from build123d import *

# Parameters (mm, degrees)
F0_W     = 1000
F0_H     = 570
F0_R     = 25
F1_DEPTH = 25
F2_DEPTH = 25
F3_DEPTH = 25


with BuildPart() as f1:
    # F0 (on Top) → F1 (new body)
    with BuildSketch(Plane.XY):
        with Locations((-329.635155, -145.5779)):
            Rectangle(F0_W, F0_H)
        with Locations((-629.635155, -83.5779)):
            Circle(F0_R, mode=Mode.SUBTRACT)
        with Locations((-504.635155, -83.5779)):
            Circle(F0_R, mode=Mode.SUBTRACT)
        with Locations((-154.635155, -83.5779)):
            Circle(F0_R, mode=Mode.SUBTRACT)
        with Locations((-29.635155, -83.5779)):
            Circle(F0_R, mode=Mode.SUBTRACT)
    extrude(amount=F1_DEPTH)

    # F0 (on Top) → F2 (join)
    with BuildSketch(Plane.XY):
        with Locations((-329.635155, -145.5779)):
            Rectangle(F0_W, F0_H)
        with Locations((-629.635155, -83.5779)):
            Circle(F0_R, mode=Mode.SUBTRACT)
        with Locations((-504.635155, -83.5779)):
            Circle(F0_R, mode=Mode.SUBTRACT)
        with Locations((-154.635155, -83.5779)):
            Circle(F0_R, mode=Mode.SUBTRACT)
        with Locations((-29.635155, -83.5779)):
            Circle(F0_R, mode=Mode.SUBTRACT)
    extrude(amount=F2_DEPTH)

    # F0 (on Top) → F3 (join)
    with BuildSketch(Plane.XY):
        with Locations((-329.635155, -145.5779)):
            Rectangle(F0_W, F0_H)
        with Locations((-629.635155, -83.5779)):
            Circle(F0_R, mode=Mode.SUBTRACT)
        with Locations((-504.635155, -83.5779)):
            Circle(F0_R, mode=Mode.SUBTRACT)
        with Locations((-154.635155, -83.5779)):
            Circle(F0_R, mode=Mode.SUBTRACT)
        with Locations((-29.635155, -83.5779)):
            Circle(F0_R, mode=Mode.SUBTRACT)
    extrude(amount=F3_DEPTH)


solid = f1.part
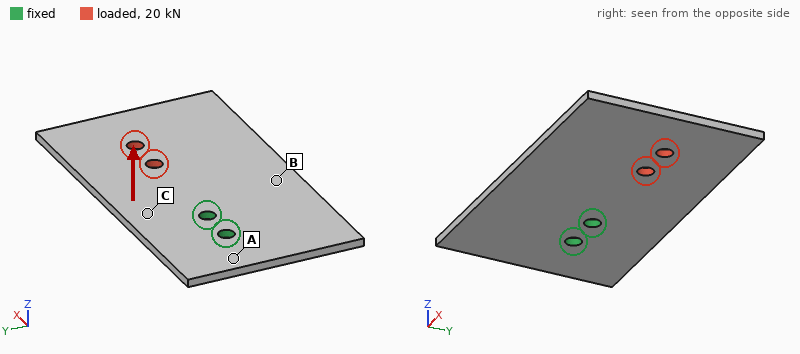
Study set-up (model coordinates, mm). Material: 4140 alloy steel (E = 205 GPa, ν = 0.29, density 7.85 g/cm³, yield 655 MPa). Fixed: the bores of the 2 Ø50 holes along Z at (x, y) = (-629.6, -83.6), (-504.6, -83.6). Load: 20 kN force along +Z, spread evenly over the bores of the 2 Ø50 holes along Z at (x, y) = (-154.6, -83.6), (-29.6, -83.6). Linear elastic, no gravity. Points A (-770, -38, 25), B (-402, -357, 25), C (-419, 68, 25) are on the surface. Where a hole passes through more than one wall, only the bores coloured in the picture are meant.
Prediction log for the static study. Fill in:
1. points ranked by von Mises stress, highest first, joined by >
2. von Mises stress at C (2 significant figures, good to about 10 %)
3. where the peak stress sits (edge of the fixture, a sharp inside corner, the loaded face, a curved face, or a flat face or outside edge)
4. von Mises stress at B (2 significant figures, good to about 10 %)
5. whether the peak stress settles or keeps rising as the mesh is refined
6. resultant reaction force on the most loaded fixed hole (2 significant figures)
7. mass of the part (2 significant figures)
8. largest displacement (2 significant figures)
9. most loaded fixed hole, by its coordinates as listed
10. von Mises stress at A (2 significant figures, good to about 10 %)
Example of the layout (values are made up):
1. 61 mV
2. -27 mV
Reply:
1. C > B > A
2. 110 MPa
3. edge of the fixture
4. 72 MPa
5. keeps rising
6. 45 kN
7. 110 kg
8. 6.9 mm
9. (-504.6, -83.6)
10. 21 MPa
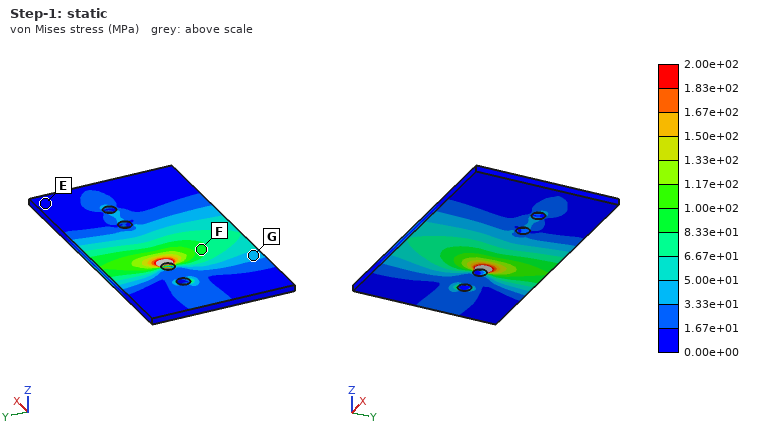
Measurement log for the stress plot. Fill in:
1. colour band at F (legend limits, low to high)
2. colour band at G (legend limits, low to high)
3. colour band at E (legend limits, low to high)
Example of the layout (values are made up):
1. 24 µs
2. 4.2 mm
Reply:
1. 8.33e+01 to 1.00e+02 MPa
2. 3.33e+01 to 5.00e+01 MPa
3. 0.00e+00 to 1.67e+01 MPa
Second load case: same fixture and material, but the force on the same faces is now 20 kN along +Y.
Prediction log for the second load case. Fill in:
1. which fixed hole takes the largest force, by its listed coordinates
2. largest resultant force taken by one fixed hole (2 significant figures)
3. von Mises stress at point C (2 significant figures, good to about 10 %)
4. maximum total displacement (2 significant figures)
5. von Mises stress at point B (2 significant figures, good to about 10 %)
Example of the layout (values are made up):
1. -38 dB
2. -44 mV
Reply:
1. (-504.6, -83.6)
2. 66 kN
3. 4.6 MPa
4. 100 µm
5. 3.2 MPa
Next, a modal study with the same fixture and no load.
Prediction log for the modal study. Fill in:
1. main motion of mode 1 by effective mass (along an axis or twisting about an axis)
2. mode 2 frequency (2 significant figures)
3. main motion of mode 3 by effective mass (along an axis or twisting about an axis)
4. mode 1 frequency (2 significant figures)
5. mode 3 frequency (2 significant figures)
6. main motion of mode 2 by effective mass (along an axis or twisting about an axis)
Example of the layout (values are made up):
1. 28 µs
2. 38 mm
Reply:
1. along Z
2. 95 Hz
3. along Z
4. 43 Hz
5. 190 Hz
6. twisting about X
